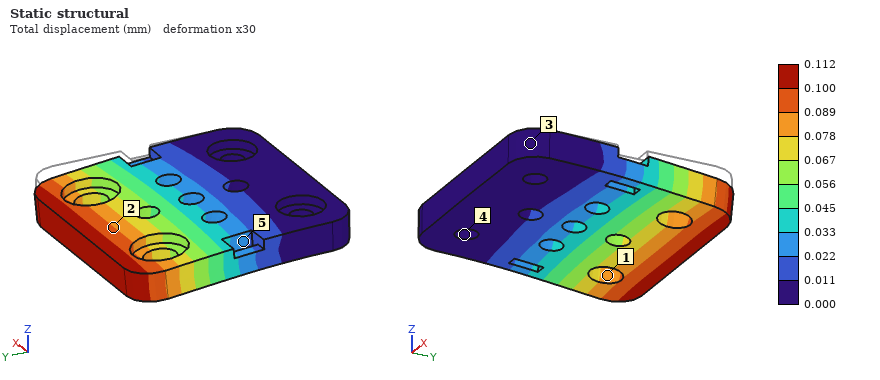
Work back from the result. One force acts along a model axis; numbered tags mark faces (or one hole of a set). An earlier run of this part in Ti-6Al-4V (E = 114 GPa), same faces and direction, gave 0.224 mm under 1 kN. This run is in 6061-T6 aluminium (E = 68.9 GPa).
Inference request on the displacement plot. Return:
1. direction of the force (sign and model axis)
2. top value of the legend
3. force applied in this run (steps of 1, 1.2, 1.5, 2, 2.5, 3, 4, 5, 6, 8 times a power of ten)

-Z
0.112 mm
300 N
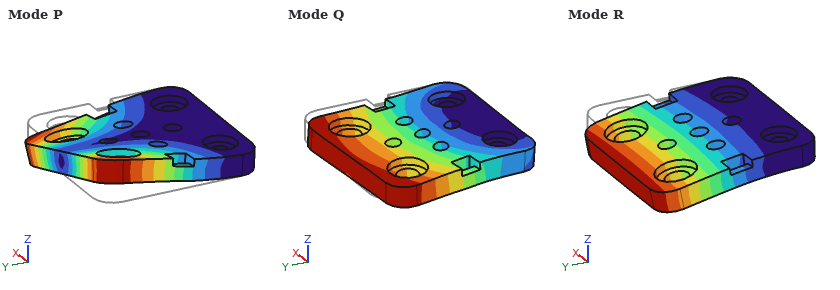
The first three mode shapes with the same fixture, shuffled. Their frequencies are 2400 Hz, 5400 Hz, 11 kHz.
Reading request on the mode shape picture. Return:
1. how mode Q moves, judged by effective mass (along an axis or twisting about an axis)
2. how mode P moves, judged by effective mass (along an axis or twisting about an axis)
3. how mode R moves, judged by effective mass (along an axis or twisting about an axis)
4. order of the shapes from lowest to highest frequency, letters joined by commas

along X
twisting about Y
along Z
R, P, Q
